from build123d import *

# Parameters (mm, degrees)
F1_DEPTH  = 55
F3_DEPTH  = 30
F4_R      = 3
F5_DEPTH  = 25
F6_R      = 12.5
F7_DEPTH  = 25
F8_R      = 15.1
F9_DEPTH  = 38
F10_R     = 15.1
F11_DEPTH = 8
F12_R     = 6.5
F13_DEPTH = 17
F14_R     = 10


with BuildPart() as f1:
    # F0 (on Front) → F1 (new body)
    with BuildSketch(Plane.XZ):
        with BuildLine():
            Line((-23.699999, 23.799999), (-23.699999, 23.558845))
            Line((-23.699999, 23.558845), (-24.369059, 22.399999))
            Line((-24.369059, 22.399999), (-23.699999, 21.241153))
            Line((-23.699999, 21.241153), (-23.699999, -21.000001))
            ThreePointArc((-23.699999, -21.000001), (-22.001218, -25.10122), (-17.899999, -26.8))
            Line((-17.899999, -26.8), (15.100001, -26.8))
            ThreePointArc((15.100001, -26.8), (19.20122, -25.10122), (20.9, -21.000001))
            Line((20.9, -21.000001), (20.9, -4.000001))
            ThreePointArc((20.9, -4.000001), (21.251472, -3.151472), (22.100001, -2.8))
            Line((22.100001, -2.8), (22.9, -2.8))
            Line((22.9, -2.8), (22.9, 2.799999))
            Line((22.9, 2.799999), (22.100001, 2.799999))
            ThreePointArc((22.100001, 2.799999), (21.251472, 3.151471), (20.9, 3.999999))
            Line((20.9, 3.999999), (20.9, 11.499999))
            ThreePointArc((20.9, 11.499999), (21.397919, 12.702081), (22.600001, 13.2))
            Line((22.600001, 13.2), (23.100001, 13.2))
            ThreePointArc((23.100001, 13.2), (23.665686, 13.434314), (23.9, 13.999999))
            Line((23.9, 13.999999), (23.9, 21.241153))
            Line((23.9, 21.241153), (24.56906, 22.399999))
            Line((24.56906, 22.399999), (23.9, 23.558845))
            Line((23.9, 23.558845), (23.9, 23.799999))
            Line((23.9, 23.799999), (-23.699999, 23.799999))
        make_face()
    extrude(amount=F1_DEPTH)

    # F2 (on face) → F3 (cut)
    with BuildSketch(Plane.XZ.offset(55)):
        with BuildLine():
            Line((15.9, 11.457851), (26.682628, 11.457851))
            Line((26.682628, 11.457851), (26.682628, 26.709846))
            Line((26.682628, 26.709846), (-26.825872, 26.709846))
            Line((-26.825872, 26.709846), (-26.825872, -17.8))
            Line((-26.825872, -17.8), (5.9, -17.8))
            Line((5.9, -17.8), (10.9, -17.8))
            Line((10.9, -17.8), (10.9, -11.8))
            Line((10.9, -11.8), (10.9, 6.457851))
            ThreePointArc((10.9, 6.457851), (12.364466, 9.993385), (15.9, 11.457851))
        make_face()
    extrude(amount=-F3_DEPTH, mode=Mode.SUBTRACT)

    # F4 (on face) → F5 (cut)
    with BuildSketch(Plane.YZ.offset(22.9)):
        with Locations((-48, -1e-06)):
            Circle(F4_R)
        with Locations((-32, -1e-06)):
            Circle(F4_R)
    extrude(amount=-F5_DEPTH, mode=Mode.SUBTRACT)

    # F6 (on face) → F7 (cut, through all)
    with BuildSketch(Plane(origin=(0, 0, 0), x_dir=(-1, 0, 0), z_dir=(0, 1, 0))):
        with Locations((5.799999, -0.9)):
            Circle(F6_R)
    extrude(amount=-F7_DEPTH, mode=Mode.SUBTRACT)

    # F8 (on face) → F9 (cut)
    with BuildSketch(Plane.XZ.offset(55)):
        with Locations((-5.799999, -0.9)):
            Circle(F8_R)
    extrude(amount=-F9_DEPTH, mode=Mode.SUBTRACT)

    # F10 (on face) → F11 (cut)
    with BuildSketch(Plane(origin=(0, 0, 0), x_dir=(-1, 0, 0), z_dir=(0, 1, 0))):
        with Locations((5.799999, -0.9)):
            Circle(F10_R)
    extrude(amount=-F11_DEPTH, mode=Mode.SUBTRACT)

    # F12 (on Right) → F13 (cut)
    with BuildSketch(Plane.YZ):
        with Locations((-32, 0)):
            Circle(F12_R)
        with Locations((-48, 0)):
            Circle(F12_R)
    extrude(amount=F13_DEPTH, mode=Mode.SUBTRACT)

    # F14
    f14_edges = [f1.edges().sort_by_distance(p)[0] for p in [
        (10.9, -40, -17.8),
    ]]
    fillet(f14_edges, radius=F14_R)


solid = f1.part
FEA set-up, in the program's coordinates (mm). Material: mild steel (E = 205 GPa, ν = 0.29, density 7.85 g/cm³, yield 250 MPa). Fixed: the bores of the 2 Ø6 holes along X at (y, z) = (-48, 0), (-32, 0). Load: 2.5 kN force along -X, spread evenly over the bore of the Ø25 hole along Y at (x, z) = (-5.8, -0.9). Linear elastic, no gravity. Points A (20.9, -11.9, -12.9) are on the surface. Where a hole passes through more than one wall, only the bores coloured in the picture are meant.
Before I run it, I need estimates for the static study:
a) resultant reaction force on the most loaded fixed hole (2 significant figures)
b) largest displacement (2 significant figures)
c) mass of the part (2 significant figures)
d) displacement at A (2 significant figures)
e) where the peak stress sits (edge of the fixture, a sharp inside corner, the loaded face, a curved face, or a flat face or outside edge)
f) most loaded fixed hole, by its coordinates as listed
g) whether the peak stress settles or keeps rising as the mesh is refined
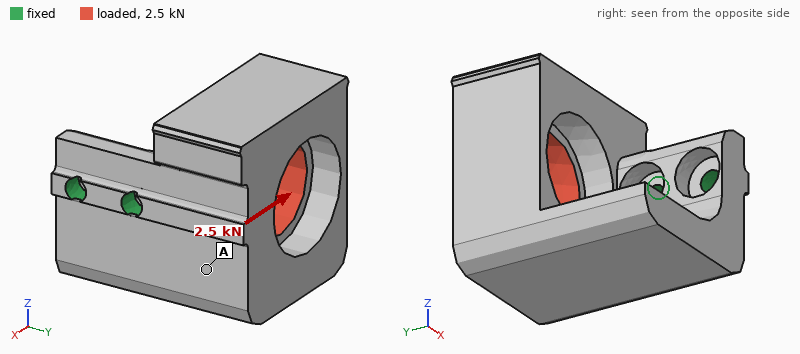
4.3 kN
48 µm
480 g
21 µm
edge of the fixture
(-32, 0)
keeps rising
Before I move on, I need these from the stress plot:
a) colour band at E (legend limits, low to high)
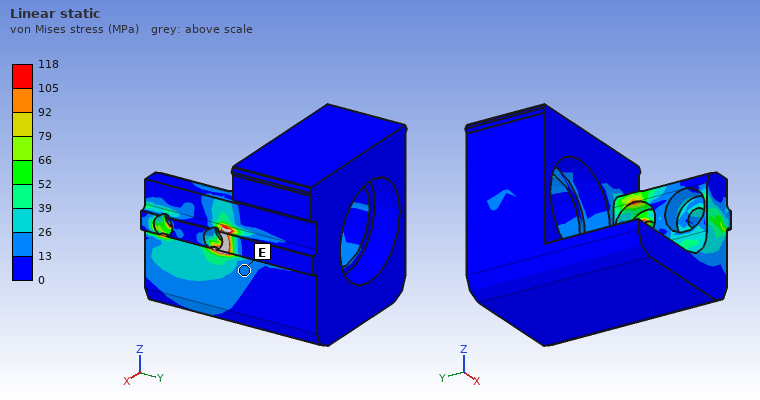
13 to 26 MPa
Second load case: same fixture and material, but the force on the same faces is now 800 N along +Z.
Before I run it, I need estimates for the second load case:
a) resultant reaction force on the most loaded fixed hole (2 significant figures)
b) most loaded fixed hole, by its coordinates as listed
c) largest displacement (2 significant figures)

1.4 kN
(-32, 0)
44 µm
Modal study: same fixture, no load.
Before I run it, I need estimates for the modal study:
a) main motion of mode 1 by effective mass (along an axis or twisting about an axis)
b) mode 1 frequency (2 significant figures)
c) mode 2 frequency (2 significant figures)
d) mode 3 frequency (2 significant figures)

along Z
1300 Hz
2000 Hz
4000 Hz
